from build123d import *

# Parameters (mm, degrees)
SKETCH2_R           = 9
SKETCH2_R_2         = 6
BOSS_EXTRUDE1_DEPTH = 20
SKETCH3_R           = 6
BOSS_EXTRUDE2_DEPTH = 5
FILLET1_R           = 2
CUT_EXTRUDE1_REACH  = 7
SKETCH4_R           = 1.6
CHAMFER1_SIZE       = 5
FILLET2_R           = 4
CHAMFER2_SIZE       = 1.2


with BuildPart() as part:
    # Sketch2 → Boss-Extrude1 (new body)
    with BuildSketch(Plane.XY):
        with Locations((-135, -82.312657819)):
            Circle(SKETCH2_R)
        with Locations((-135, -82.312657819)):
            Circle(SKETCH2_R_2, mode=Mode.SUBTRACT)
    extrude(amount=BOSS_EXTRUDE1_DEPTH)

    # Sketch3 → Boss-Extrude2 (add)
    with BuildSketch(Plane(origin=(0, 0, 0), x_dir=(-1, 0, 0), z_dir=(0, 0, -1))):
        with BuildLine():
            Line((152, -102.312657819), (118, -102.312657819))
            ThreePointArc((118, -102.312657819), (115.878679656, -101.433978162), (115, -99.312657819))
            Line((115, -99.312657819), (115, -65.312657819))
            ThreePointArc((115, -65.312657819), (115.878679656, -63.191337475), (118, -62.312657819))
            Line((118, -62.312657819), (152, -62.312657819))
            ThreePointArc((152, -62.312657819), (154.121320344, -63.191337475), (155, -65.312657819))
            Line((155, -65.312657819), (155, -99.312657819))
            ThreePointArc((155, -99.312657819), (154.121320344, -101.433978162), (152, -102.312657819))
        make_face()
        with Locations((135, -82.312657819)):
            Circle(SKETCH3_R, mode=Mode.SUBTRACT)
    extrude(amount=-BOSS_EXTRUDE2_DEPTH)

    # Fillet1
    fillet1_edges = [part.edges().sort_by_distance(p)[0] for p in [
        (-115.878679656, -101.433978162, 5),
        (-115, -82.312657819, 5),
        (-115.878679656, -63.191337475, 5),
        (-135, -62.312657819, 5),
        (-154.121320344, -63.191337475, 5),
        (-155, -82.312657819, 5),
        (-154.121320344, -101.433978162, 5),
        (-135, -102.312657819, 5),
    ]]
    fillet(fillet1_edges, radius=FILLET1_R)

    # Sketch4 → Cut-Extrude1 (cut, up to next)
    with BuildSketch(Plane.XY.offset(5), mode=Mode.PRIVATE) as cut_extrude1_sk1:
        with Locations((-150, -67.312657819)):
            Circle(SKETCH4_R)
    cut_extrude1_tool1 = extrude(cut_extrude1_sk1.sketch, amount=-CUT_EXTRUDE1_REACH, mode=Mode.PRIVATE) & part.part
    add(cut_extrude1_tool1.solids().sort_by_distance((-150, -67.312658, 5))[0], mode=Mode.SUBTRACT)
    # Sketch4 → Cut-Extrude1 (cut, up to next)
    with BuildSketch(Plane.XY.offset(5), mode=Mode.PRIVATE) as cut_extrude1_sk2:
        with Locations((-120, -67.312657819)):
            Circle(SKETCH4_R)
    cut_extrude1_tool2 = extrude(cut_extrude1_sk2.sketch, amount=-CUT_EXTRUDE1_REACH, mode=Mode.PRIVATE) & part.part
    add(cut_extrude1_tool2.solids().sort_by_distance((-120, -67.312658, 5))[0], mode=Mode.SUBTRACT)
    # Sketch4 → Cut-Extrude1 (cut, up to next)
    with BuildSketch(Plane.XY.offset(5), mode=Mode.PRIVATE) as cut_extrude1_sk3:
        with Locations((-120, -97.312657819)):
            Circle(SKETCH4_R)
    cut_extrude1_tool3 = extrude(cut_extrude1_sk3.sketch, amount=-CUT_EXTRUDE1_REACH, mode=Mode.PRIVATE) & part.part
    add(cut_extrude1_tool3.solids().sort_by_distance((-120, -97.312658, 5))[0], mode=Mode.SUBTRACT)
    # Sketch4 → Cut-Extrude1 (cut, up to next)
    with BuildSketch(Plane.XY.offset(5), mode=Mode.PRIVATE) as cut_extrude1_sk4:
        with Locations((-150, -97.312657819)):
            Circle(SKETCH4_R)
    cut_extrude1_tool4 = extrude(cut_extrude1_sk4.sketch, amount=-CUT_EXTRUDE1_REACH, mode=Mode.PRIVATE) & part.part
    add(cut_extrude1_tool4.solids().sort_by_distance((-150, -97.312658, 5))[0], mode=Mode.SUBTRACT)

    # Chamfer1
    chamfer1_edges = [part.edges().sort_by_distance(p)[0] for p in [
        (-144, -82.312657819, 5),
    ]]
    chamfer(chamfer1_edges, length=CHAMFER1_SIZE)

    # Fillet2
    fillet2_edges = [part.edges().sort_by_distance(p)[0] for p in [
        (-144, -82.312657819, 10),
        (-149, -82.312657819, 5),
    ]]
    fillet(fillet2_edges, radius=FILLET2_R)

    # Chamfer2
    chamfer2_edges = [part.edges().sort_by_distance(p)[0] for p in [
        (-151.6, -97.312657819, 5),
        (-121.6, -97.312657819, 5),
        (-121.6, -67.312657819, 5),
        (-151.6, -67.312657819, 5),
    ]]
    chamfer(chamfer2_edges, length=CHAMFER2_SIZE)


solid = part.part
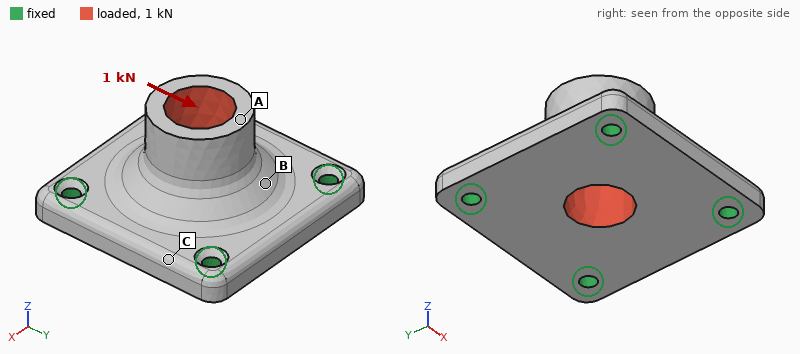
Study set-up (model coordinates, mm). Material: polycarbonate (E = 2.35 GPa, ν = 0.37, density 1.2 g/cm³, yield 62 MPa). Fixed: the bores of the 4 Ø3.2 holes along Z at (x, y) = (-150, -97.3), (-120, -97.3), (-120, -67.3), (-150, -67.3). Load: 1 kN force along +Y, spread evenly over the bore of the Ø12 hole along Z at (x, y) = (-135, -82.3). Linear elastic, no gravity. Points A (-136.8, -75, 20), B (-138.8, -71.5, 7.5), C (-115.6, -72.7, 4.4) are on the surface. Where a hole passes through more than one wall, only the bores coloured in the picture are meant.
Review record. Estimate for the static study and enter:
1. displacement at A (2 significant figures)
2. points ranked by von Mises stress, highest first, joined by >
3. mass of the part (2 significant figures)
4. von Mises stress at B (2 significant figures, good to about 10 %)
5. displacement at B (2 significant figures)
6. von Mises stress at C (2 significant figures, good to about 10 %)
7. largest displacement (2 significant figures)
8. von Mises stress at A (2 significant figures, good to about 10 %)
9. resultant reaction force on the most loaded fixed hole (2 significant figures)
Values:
0.19 mm
B > A > C
12 g
7.3 MPa
0.079 mm
2.1 MPa
0.19 mm
5.1 MPa
320 N
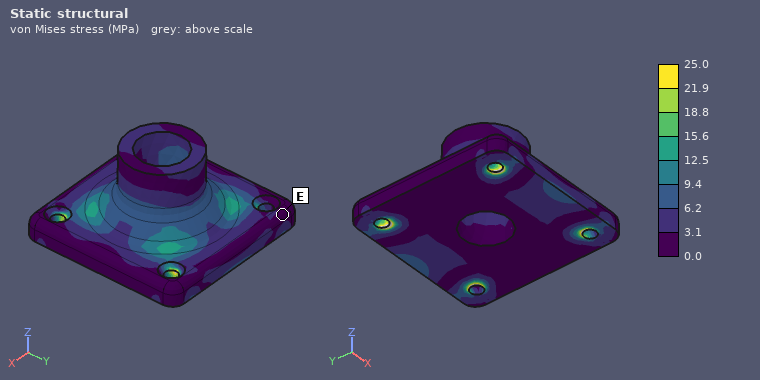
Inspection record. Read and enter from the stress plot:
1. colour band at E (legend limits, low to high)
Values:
0.0 to 3.1 MPa
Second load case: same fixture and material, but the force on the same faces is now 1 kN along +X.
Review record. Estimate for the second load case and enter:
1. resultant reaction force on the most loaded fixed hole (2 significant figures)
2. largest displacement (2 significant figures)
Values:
320 N
0.19 mm
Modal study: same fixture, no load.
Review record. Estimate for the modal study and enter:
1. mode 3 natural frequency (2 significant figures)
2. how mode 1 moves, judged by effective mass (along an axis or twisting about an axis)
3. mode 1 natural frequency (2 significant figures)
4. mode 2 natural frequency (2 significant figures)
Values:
5700 Hz
along Z
4700 Hz
5700 Hz
